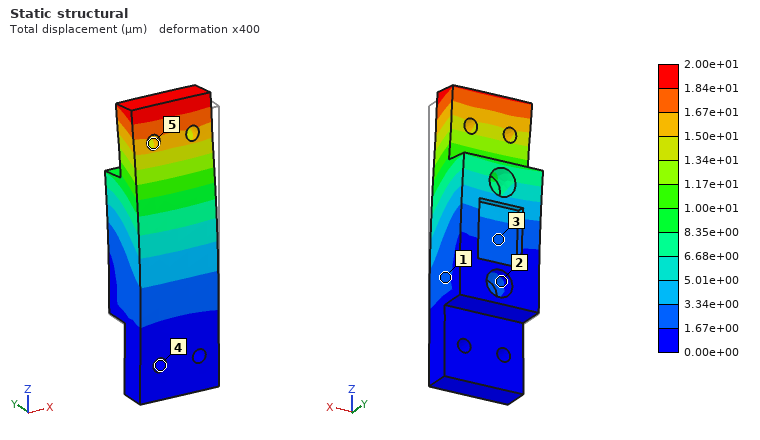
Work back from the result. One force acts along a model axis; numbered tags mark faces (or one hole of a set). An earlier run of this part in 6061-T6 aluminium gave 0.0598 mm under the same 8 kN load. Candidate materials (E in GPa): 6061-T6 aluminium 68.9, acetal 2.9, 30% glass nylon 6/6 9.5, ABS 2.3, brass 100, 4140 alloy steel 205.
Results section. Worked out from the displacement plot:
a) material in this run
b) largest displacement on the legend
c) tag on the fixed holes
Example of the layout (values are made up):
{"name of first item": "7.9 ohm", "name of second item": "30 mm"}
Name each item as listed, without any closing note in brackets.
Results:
{"material in this run": "4140 alloy steel", "largest displacement on the legend": "2.00e+01 µm", "tag on the fixed holes": "4"}
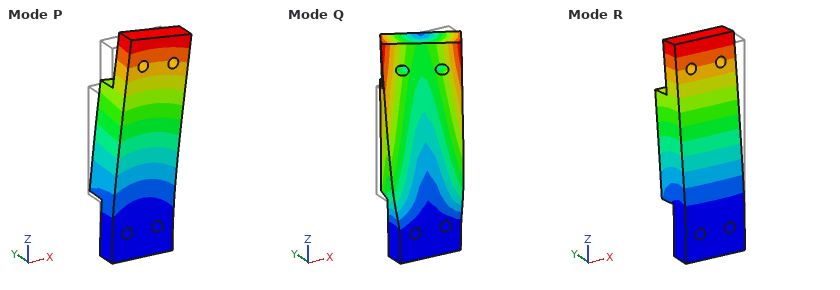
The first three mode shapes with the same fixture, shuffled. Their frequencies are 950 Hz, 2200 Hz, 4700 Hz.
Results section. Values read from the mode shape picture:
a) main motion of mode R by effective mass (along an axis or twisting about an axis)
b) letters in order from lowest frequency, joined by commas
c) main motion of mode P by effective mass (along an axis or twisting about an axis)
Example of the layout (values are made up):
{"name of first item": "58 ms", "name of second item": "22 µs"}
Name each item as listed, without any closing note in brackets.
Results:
{"main motion of mode R by effective mass": "along Y", "letters in order from lowest frequency, joined by commas": "R, P, Q", "main motion of mode P by effective mass": "along X"}
